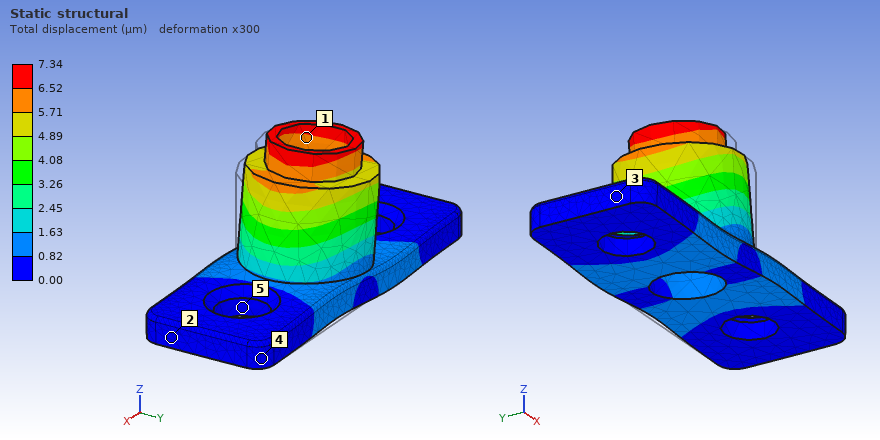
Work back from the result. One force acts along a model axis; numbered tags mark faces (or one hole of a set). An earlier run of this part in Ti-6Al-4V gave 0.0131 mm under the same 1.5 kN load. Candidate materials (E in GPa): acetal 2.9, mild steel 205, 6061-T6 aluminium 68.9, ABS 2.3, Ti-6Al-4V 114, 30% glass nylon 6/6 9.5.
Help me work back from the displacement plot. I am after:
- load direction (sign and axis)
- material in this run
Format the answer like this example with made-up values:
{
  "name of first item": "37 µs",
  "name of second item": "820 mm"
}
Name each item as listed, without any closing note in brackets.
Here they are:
{
  "load direction": "-X",
  "material in this run": "mild steel"
}
